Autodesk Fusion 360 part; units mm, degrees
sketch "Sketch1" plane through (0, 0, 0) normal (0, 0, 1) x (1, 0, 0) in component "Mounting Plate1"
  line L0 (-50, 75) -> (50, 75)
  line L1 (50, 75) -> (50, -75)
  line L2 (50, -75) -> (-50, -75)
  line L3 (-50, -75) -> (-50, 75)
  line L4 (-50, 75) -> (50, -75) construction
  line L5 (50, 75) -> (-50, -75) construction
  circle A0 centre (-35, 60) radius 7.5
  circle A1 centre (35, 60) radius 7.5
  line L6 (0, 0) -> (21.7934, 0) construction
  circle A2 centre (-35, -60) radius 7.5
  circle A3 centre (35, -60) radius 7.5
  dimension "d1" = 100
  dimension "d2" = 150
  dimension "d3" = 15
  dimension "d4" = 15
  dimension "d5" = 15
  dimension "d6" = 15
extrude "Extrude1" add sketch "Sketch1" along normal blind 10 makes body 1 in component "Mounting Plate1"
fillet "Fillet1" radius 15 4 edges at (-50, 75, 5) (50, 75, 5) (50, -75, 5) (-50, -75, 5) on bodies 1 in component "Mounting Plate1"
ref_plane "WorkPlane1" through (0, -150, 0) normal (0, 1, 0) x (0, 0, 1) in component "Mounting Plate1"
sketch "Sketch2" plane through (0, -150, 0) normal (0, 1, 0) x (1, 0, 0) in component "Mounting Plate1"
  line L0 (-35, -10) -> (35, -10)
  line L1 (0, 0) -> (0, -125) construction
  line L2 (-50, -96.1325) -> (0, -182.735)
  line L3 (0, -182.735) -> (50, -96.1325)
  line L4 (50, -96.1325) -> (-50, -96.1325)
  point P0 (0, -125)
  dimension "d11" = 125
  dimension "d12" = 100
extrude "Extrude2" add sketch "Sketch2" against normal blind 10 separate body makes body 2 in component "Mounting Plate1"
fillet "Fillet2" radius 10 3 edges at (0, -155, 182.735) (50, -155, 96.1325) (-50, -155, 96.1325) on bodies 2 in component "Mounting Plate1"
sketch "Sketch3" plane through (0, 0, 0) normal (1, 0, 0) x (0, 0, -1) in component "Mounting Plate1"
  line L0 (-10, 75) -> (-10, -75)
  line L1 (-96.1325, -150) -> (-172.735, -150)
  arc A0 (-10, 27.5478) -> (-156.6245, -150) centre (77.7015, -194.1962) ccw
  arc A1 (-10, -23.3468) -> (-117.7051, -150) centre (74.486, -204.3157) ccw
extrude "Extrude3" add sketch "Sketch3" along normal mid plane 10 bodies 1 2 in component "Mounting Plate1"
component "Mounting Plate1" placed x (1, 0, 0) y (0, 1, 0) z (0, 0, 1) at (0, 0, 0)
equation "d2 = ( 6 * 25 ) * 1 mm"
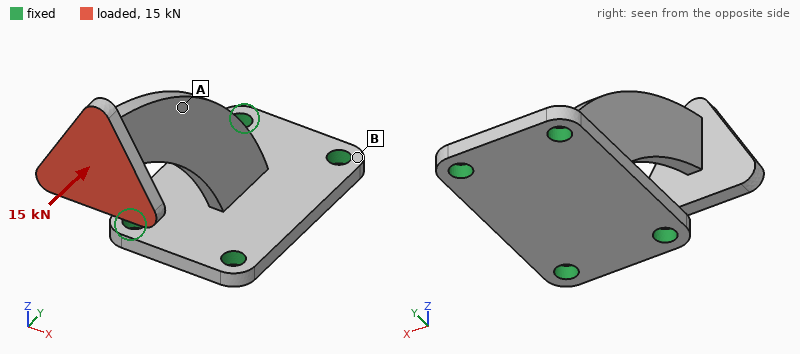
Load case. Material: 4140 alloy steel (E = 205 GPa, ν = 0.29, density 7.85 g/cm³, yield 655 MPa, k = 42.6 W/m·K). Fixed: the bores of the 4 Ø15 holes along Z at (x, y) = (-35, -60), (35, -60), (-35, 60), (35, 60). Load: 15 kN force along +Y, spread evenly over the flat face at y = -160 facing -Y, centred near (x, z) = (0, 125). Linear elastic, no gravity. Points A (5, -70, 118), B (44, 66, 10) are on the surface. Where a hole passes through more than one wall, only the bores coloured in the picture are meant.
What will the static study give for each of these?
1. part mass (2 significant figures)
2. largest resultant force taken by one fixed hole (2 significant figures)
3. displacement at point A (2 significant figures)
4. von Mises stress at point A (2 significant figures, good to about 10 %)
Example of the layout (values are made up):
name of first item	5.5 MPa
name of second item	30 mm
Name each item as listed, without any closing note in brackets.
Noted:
part mass	2.1 kg
largest resultant force taken by one fixed hole	12 kN
displacement at point A	1.3 mm
von Mises stress at point A	99 MPa
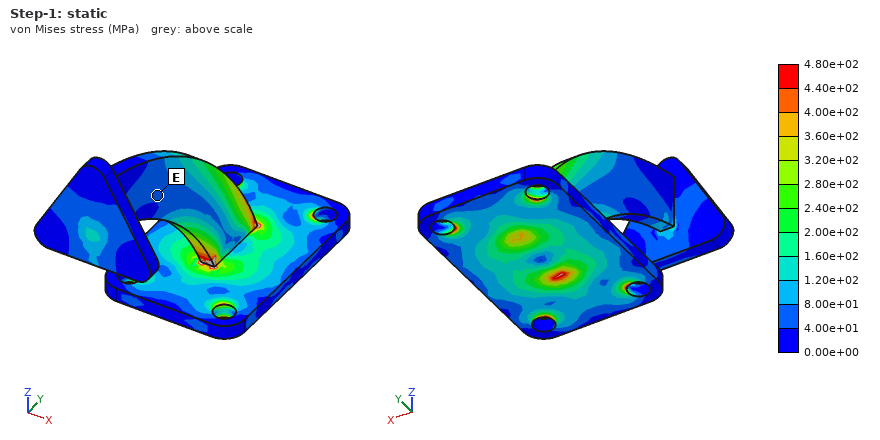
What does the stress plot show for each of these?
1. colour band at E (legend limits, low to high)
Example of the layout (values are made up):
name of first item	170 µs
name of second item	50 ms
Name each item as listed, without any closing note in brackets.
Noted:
colour band at E	4.00e+01 to 8.00e+01 MPa
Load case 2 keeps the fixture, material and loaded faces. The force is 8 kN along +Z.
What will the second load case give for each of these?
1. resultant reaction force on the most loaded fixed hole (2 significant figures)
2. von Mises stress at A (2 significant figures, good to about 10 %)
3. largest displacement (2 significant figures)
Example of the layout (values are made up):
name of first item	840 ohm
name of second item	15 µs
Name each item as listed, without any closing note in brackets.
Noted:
resultant reaction force on the most loaded fixed hole	9.4 kN
von Mises stress at A	140 MPa
largest displacement	2.5 mm
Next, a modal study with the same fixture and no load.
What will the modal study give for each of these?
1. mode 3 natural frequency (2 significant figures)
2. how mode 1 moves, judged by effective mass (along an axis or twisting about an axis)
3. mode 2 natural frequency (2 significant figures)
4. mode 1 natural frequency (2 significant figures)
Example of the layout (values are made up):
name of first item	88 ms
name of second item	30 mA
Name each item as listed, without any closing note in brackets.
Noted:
mode 3 natural frequency	570 Hz
how mode 1 moves, judged by effective mass	along X
mode 2 natural frequency	420 Hz
mode 1 natural frequency	130 Hz
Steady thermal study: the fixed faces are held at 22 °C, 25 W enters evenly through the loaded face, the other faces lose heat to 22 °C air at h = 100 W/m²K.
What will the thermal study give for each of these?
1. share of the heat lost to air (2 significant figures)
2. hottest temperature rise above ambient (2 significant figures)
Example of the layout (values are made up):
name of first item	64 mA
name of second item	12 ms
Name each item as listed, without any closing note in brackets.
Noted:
share of the heat lost to air	100 %
hottest temperature rise above ambient	27 K
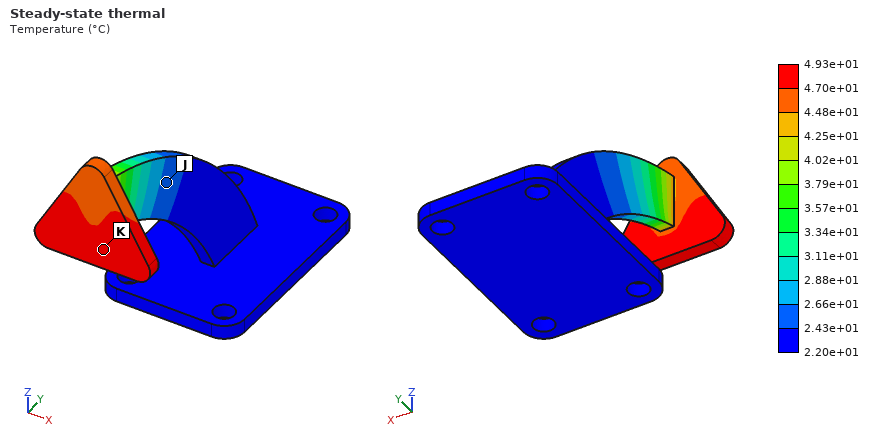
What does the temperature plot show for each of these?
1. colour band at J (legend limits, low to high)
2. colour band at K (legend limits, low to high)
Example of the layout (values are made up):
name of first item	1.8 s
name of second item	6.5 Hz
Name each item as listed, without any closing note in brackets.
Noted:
colour band at J	2.43e+01 to 2.66e+01 °C
colour band at K	4.70e+01 to 4.93e+01 °C
